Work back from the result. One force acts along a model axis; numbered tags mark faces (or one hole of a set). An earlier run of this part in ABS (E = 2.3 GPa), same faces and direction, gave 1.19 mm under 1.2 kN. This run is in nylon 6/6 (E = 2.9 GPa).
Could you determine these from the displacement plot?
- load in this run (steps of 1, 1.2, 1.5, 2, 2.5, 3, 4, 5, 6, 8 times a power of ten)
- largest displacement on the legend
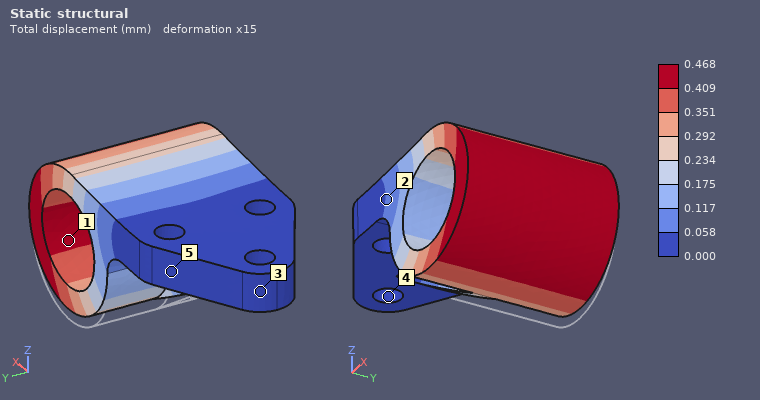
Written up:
600 N
0.468 mm
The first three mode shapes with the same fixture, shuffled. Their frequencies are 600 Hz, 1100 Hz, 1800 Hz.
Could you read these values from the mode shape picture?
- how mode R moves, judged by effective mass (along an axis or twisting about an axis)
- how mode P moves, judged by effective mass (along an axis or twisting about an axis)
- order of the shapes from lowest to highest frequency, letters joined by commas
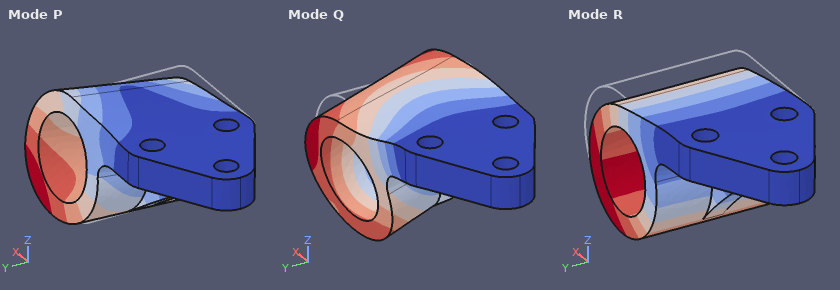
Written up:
along Z
along Y
R, P, Q
